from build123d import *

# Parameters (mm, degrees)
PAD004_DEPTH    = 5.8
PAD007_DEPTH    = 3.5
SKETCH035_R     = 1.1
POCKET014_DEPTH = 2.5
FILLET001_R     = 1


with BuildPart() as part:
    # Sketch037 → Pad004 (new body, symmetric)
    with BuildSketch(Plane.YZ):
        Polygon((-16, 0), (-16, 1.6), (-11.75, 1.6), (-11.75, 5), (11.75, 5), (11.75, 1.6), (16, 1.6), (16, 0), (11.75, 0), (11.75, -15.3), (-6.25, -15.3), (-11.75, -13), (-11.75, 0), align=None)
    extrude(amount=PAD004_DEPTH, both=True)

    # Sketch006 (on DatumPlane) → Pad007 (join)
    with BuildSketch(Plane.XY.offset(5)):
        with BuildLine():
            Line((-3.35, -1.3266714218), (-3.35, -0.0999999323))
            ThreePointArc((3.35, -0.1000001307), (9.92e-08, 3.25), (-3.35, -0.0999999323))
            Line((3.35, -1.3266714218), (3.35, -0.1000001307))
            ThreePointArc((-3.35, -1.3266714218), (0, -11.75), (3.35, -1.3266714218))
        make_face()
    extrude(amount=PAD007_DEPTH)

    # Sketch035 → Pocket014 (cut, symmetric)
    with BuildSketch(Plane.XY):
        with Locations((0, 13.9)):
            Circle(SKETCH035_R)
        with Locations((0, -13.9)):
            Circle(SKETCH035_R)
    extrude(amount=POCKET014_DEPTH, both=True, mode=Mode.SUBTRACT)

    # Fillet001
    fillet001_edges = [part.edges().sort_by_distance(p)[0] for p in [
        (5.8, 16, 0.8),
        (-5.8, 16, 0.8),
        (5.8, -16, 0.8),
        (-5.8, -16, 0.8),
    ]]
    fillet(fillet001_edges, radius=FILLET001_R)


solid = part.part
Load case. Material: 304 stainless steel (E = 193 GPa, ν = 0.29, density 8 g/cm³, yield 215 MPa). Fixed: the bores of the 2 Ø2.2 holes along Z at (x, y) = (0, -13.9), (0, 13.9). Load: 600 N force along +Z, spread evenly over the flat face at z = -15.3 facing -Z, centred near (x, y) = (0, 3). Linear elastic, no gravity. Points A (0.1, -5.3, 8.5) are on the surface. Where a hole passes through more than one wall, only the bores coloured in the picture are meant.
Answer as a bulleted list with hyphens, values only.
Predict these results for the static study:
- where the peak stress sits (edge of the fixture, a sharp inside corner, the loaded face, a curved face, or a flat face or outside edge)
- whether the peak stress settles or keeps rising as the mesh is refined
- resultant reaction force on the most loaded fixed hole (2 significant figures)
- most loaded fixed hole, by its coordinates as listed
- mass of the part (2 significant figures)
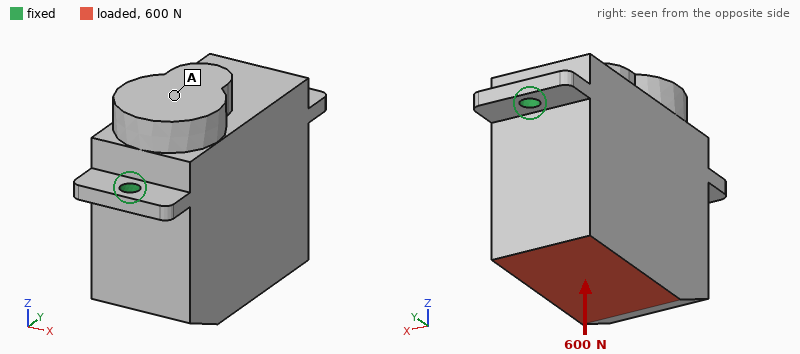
- edge of the fixture
- keeps rising
- 370 N
- (0, 13.9)
- 48 g
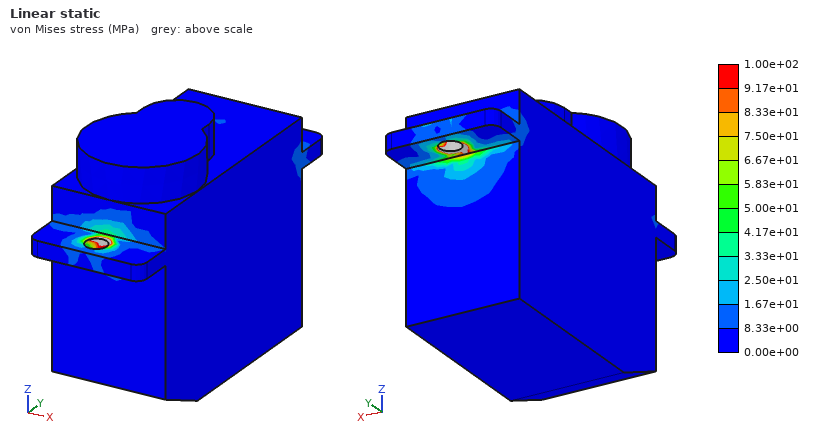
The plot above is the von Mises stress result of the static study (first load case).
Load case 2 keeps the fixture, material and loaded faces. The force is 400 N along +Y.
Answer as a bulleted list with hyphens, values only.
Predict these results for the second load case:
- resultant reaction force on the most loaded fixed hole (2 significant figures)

- 330 N
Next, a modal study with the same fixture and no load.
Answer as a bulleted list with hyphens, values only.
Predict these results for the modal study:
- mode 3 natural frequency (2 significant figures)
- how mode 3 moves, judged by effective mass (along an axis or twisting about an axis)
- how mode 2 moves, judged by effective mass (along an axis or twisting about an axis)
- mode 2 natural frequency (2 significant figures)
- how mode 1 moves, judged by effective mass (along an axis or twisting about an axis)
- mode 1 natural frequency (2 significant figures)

- 15 kHz
- along Y
- along Z
- 13 kHz
- along X
- 2900 Hz
